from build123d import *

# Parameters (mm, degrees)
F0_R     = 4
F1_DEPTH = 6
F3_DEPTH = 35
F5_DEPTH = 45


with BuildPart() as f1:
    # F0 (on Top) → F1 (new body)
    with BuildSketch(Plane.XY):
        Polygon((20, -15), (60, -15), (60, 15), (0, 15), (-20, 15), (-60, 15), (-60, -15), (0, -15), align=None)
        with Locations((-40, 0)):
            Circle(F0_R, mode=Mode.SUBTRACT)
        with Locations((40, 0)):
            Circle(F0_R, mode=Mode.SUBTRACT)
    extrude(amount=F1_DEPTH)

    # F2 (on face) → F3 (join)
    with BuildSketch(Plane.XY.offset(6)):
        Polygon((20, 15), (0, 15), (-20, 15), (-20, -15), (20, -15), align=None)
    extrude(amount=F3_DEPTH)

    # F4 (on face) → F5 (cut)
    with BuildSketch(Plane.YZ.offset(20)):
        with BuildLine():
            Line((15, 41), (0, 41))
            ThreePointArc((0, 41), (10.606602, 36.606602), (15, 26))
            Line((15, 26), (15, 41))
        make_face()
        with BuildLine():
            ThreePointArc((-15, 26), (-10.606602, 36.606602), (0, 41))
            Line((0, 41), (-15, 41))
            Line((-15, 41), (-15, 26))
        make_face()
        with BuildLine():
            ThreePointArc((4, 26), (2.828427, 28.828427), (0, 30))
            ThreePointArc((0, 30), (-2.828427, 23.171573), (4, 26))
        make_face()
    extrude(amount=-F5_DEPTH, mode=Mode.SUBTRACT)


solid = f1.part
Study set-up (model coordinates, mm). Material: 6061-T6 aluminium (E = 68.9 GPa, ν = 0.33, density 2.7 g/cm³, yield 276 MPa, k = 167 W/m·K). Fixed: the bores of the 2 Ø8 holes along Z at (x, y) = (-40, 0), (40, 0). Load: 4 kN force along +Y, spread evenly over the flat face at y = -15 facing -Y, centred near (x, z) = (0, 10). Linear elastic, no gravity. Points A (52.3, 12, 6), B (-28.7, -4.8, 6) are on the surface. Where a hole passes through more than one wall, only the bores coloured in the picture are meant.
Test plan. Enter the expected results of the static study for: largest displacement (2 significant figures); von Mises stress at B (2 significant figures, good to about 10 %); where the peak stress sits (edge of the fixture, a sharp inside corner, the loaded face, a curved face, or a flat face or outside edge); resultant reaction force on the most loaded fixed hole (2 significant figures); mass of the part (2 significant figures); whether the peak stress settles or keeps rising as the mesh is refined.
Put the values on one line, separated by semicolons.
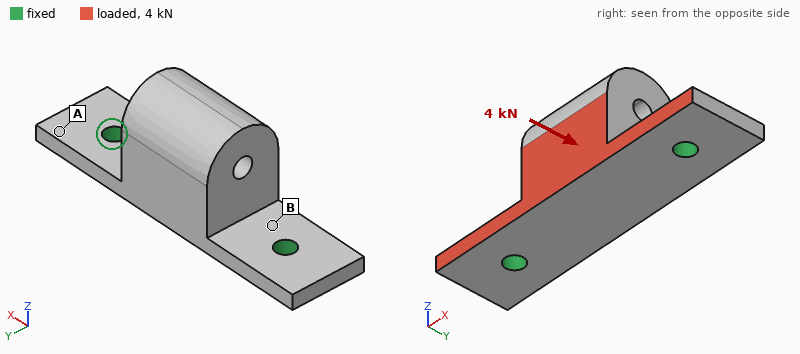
0.18 mm; 68 MPa; edge of the fixture; 2.0 kN; 150 g; keeps rising
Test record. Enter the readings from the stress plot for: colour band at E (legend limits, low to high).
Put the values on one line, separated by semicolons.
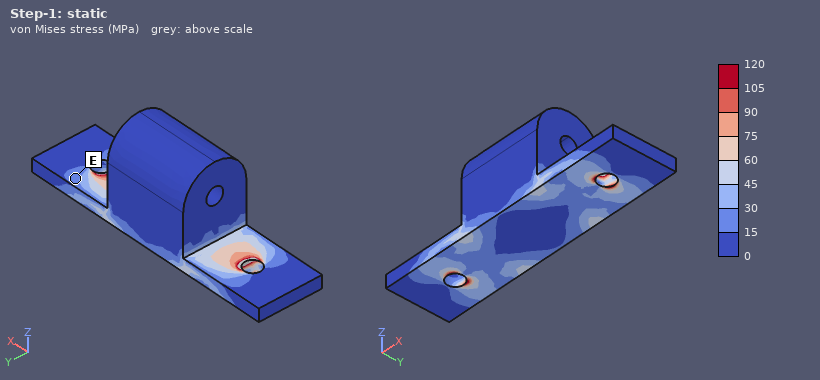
15 to 30 MPa
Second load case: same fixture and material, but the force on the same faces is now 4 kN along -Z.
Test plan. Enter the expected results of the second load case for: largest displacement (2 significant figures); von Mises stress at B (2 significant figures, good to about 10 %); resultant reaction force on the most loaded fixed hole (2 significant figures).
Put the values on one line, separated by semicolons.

0.27 mm; 77 MPa; 2.1 kN
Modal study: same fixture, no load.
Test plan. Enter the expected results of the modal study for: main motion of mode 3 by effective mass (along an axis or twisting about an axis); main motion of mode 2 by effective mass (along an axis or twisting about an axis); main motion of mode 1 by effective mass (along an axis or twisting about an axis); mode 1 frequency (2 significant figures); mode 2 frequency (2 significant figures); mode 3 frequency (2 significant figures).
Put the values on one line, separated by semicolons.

along X; along Z; along Y; 1700 Hz; 3700 Hz; 4700 Hz
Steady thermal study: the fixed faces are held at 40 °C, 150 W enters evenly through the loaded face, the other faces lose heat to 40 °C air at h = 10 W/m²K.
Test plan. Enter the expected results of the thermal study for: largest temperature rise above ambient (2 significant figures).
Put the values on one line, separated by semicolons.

55 K
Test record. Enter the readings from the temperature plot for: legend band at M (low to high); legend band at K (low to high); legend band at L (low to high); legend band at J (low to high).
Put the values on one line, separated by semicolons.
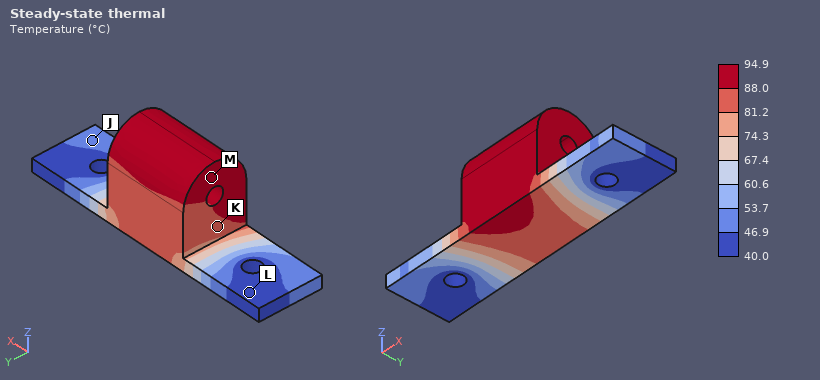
88.0 to 94.9 °C; 81.2 to 88.0 °C; 40.0 to 46.9 °C; 46.9 to 53.7 °C
